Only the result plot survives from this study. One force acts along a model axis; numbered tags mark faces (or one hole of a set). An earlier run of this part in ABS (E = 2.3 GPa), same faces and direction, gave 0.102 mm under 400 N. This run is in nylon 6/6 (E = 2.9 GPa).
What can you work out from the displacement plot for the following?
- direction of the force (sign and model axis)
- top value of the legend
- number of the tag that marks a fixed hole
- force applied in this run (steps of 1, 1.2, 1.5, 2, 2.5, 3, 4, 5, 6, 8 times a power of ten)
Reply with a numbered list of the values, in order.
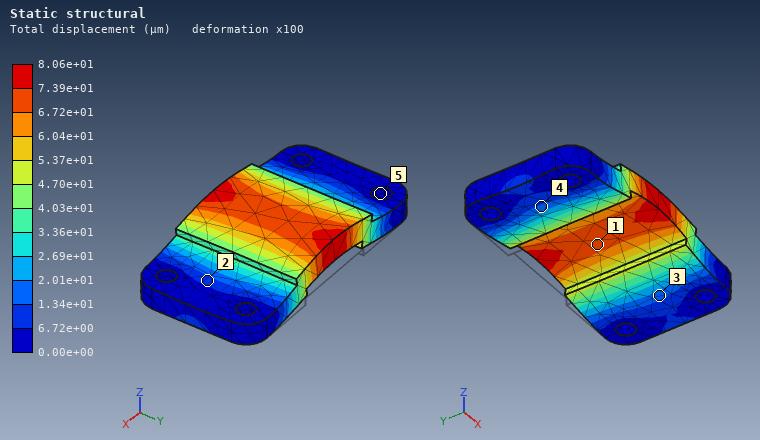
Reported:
1. +Z
2. 8.06e+01 µm
3. 5
4. 400 N
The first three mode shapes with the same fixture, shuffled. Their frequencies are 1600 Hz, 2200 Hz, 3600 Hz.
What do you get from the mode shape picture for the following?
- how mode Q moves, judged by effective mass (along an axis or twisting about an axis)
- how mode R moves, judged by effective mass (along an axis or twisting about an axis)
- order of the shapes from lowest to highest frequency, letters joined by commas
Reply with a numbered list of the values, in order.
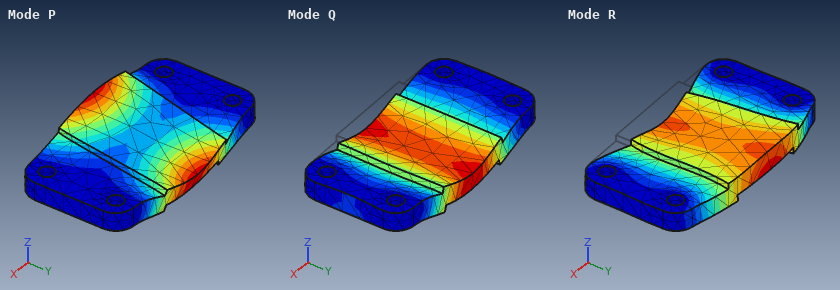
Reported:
1. along Z
2. along Y
3. Q, P, R
